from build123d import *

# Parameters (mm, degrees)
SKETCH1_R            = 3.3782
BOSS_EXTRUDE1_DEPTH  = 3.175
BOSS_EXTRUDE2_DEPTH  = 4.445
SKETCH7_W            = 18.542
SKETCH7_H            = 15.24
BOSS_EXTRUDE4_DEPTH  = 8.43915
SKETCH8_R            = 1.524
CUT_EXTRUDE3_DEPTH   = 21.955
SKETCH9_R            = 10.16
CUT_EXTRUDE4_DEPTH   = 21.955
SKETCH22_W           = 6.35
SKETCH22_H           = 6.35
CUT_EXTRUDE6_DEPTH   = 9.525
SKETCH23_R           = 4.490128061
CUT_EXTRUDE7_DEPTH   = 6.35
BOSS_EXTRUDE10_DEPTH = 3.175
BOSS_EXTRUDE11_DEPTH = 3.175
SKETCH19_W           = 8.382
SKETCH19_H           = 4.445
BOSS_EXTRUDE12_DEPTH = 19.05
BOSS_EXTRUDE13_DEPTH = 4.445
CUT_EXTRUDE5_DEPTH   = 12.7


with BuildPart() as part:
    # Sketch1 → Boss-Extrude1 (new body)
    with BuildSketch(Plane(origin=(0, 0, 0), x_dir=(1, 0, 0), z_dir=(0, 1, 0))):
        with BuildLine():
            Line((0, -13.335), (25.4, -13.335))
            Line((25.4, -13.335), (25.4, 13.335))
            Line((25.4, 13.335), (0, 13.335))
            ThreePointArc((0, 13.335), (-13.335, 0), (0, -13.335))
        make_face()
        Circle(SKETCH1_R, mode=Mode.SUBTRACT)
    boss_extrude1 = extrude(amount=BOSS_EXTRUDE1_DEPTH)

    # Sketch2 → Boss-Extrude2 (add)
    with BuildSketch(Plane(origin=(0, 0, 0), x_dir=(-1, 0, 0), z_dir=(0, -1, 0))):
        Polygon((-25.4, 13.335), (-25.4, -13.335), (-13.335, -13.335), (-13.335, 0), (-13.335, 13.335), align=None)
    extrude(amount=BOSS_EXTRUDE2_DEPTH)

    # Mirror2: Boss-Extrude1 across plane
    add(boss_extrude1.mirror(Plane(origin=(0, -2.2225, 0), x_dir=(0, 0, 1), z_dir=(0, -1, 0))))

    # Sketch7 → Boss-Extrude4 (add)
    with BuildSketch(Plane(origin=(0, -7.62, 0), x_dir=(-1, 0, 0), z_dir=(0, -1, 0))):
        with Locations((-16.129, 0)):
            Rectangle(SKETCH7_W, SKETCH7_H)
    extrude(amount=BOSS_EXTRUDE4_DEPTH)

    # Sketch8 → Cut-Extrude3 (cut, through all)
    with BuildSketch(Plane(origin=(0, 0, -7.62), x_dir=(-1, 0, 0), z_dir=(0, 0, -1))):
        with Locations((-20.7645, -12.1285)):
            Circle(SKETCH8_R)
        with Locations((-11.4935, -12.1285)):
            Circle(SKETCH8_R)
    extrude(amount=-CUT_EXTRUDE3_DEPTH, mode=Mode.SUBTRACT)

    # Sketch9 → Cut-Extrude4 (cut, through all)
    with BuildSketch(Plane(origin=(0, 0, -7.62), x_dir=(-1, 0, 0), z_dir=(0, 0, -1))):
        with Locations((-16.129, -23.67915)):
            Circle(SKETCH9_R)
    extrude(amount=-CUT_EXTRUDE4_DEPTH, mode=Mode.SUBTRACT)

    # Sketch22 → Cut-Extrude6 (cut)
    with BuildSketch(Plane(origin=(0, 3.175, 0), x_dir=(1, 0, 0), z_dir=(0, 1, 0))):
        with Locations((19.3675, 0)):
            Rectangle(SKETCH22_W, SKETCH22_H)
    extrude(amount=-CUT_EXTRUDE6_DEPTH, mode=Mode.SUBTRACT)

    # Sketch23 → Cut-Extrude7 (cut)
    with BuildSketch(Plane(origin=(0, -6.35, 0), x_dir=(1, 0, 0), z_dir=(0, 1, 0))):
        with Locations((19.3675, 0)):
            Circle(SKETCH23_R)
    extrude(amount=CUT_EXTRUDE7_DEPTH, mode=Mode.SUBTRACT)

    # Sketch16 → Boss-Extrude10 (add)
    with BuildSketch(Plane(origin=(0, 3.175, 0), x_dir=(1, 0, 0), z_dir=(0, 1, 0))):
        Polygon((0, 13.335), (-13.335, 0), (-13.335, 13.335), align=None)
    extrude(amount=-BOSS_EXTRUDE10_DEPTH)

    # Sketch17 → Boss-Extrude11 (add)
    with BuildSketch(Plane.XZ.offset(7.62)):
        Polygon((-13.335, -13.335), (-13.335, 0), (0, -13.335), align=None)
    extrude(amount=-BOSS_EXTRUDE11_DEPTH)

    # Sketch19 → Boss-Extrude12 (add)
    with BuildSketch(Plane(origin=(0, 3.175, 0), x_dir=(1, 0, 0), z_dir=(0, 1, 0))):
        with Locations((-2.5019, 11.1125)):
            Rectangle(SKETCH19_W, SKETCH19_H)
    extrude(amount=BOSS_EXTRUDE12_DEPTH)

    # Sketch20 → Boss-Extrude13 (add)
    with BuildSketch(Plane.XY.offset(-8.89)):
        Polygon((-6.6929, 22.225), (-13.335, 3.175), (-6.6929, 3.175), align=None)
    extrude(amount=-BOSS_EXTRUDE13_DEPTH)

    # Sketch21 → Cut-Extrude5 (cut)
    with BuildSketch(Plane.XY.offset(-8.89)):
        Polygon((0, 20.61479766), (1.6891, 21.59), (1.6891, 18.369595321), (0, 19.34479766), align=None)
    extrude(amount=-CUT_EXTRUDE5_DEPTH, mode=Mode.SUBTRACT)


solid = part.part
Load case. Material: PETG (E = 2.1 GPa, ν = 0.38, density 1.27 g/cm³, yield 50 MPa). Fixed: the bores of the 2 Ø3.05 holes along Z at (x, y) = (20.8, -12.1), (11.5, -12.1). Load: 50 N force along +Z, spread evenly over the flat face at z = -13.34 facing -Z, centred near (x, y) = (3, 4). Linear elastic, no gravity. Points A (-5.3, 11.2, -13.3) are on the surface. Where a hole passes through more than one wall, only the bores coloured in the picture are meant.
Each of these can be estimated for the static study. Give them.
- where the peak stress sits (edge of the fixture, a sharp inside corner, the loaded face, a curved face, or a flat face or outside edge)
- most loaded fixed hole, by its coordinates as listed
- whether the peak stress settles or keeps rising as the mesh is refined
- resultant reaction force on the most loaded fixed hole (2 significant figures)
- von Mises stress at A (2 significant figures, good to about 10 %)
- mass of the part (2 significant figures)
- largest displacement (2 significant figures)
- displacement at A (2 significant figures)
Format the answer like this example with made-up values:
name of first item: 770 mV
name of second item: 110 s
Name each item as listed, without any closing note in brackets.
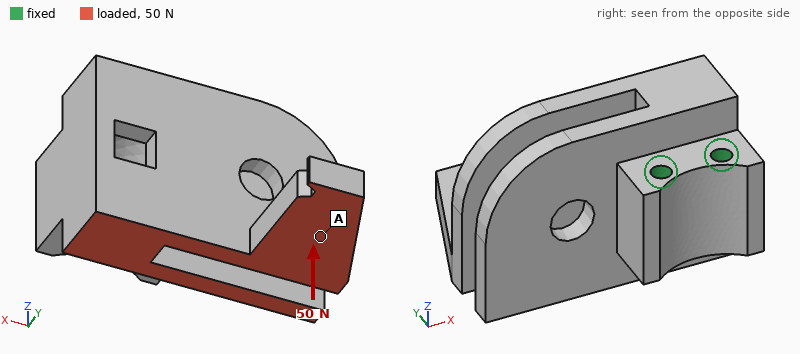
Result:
where the peak stress sits: a sharp inside corner
most loaded fixed hole, by its coordinates as listed: (11.5, -12.1)
whether the peak stress settles or keeps rising as the mesh is refined: keeps rising
resultant reaction force on the most loaded fixed hole: 57 N
von Mises stress at A: 1.3 MPa
mass of the part: 12 g
largest displacement: 0.61 mm
displacement at A: 0.34 mm
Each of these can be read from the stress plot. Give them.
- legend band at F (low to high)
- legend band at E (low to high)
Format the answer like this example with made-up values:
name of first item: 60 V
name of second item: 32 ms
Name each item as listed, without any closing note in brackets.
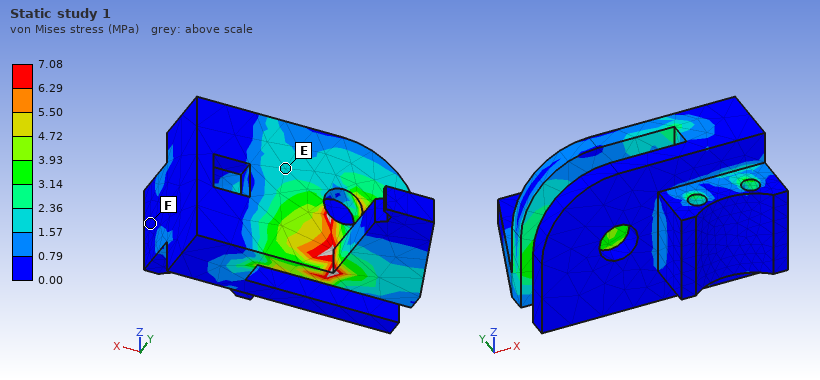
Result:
legend band at F: 0.00 to 0.79 MPa
legend band at E: 1.57 to 2.36 MPa
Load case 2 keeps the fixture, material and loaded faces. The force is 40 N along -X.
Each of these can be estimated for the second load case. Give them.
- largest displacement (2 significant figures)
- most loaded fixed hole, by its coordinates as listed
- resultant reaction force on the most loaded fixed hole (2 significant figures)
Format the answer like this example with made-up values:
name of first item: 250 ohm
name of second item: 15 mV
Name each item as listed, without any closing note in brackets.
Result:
largest displacement: 0.67 mm
most loaded fixed hole, by its coordinates as listed: (11.5, -12.1)
resultant reaction force on the most loaded fixed hole: 65 N
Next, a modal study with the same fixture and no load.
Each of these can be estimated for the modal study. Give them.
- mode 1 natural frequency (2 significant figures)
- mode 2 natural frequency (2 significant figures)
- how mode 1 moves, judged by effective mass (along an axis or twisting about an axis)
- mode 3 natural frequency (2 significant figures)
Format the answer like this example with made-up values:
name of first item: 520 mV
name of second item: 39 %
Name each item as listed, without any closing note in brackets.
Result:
mode 1 natural frequency: 550 Hz
mode 2 natural frequency: 1000 Hz
how mode 1 moves, judged by effective mass: along Y
mode 3 natural frequency: 1400 Hz
